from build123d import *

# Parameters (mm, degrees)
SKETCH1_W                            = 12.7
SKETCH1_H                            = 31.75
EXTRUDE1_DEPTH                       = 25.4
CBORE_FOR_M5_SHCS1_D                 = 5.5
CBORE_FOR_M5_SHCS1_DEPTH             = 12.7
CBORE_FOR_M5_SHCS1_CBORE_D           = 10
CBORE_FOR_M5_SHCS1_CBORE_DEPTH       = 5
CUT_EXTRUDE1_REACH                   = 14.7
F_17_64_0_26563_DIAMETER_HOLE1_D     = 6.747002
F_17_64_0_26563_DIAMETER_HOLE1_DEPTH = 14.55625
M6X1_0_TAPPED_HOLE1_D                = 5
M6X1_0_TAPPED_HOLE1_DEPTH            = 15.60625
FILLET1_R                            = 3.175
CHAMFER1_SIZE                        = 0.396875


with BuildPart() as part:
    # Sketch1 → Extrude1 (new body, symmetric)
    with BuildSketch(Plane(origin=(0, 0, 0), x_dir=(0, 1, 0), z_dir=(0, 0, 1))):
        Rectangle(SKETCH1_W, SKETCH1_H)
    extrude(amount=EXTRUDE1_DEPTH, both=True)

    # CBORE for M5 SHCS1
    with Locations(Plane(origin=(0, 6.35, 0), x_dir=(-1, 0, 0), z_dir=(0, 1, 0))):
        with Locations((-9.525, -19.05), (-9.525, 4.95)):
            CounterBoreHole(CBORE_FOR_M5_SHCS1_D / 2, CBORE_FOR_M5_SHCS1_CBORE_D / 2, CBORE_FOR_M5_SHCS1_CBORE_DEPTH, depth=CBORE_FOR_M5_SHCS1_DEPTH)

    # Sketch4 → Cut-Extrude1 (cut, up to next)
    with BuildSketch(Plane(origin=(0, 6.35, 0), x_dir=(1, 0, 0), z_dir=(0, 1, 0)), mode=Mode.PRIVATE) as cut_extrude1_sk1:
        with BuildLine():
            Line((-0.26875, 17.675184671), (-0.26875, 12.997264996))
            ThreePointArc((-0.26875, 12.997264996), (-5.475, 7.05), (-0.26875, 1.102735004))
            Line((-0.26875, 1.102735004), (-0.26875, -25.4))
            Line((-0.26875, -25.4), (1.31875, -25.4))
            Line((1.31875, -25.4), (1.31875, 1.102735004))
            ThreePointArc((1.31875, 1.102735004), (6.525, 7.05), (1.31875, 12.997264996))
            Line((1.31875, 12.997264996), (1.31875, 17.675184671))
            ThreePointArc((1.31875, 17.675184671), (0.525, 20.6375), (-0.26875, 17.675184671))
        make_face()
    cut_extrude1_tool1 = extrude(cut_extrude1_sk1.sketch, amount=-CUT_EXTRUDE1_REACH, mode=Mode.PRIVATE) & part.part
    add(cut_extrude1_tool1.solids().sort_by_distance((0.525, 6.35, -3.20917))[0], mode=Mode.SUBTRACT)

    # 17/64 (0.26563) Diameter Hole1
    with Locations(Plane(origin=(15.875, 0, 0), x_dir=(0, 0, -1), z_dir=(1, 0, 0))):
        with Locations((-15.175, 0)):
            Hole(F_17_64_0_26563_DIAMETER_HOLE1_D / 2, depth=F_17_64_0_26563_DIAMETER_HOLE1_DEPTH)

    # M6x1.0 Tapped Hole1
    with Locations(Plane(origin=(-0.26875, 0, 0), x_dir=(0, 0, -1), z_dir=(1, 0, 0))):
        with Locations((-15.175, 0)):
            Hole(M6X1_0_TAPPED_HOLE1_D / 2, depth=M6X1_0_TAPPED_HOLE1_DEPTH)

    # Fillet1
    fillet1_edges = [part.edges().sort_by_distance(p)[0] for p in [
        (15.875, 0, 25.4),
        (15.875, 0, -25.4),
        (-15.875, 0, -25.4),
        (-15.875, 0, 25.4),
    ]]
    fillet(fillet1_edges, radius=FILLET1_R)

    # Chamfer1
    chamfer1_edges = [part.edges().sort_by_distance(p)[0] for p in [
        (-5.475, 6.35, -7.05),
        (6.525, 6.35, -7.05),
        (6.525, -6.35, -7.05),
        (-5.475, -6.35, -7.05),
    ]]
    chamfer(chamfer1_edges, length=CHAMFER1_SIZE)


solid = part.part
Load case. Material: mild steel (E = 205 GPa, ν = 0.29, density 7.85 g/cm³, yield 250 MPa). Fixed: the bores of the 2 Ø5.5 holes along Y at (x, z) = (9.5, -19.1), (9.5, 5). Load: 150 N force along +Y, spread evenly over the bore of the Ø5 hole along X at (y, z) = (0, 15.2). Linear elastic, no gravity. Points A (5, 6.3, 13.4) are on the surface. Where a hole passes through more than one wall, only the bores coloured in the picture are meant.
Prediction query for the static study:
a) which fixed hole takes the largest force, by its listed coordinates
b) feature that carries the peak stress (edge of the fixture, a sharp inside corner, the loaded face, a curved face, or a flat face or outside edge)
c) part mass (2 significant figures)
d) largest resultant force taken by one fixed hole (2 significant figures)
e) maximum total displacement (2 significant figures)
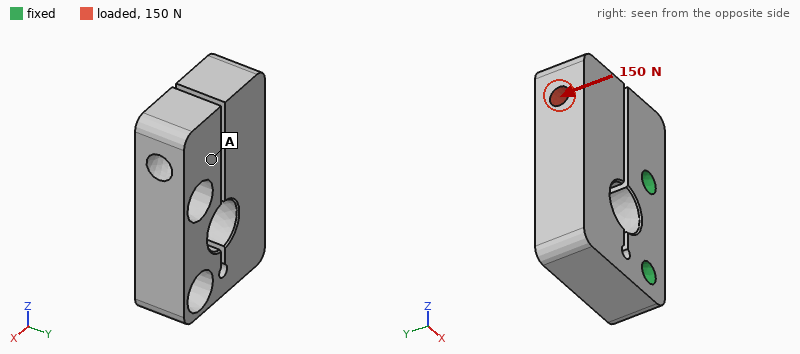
(9.5, 5)
a curved face
130 g
110 N
54 µm
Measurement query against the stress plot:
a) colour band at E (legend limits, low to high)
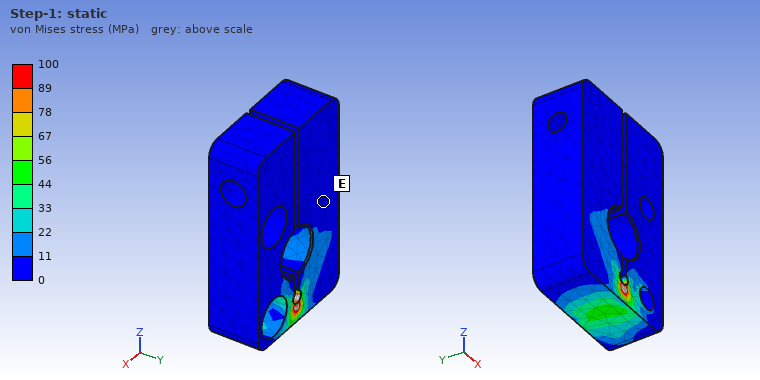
0 to 11 MPa
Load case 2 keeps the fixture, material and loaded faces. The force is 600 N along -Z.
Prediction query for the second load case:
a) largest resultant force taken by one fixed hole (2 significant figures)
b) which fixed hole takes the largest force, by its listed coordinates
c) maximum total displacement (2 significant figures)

540 N
(9.5, -19.1)
86 µm
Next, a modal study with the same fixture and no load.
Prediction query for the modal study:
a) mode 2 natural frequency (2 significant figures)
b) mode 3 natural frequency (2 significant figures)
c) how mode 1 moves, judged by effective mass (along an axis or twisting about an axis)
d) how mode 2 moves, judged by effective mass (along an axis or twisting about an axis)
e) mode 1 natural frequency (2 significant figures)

1600 Hz
6100 Hz
along X
along Y
1100 Hz
